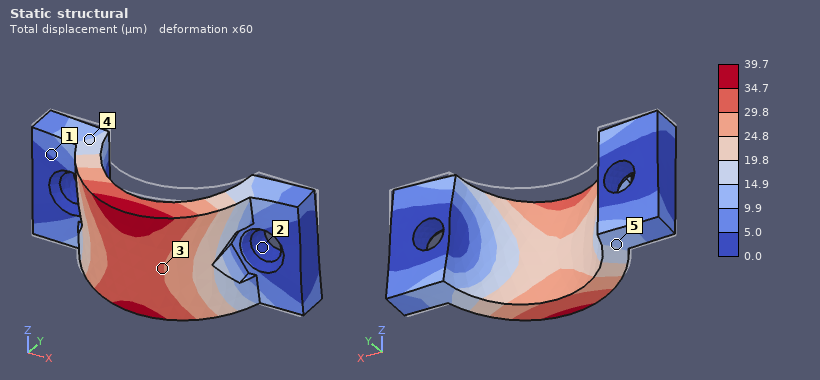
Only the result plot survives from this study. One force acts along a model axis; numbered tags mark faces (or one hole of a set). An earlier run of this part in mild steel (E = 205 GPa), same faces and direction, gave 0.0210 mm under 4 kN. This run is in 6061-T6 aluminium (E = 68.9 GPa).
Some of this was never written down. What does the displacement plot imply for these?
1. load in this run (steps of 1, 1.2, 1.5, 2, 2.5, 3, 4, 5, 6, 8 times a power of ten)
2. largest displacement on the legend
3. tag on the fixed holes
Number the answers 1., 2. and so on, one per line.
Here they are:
1. 2.5 kN
2. 39.7 µm
3. 2
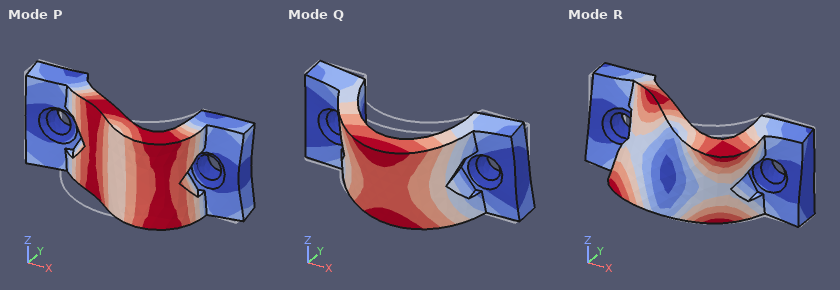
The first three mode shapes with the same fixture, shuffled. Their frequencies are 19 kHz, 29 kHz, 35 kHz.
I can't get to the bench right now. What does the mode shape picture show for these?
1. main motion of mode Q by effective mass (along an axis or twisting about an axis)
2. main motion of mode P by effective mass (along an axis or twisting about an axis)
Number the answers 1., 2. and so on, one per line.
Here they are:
1. along Z
2. along X
